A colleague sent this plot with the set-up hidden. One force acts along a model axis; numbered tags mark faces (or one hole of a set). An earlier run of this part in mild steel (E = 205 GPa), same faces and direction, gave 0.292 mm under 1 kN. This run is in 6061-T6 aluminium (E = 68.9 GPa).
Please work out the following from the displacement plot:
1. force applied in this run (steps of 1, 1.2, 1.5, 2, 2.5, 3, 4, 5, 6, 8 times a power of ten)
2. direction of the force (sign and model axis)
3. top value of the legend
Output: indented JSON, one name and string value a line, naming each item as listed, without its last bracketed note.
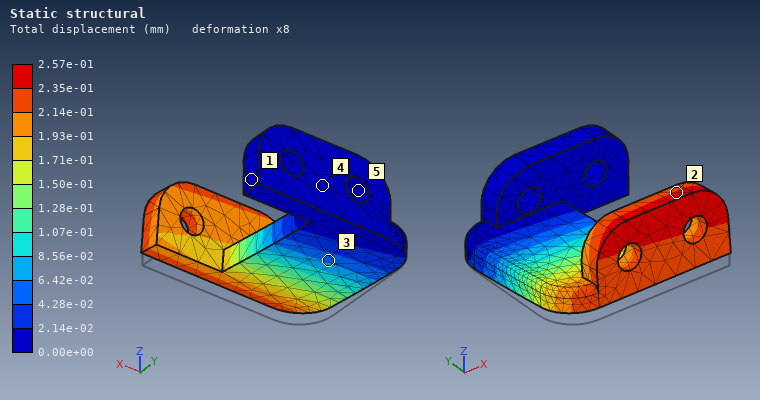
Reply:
{
  "force applied in this run": "300 N",
  "direction of the force": "+Z",
  "top value of the legend": "2.57e-01 mm"
}
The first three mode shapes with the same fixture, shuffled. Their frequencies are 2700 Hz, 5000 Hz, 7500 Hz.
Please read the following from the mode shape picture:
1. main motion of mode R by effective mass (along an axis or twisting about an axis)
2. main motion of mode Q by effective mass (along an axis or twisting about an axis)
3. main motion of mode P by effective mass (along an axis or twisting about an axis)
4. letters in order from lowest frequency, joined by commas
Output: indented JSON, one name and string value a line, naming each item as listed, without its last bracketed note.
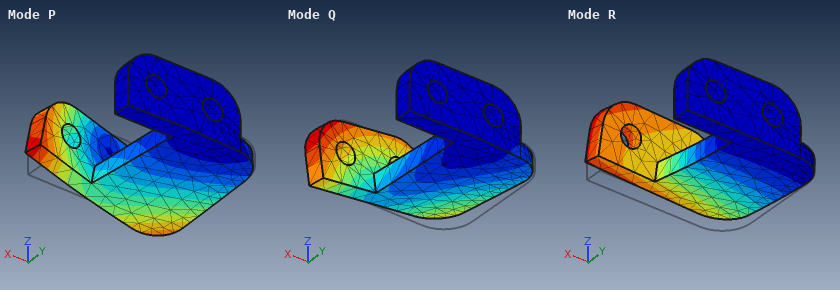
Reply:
{
  "main motion of mode R by effective mass": "along Z",
  "main motion of mode Q by effective mass": "along X",
  "main motion of mode P by effective mass": "along X",
  "letters in order from lowest frequency, joined by commas": "R, Q, P"
}
